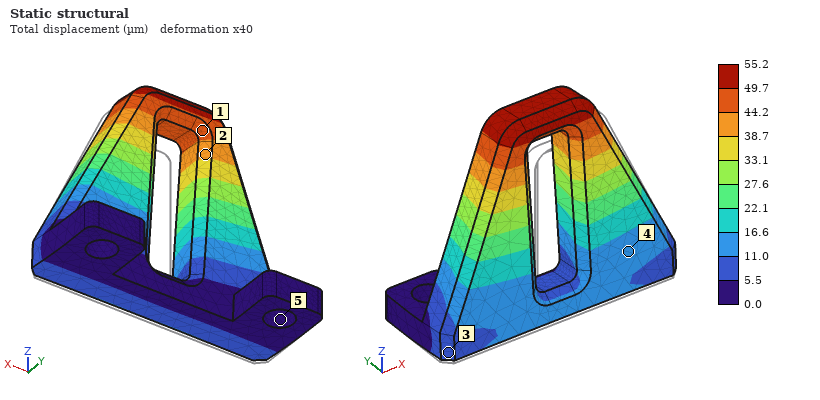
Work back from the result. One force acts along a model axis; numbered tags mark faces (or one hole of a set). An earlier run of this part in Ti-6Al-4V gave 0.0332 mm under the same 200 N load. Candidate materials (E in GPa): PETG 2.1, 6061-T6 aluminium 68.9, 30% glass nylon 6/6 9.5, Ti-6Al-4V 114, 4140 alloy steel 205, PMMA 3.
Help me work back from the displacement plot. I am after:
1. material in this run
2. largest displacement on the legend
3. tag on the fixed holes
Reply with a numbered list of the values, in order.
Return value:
1. 6061-T6 aluminium
2. 55.2 µm
3. 5
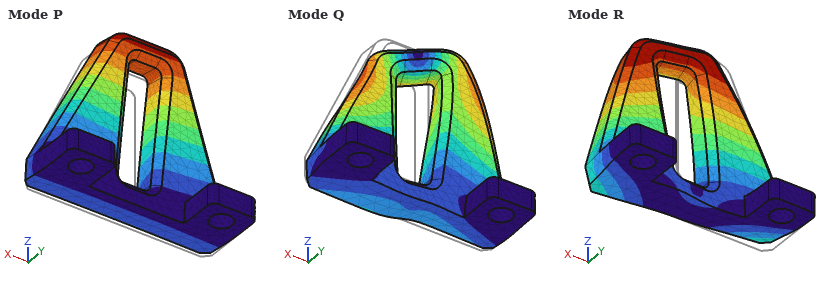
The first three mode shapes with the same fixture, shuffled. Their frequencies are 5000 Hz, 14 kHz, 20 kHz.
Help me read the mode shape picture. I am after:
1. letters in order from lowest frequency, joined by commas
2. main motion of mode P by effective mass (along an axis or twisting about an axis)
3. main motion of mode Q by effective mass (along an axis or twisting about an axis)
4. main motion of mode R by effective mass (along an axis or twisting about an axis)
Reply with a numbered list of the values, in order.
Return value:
1. P, R, Q
2. along Y
3. along X
4. along X
